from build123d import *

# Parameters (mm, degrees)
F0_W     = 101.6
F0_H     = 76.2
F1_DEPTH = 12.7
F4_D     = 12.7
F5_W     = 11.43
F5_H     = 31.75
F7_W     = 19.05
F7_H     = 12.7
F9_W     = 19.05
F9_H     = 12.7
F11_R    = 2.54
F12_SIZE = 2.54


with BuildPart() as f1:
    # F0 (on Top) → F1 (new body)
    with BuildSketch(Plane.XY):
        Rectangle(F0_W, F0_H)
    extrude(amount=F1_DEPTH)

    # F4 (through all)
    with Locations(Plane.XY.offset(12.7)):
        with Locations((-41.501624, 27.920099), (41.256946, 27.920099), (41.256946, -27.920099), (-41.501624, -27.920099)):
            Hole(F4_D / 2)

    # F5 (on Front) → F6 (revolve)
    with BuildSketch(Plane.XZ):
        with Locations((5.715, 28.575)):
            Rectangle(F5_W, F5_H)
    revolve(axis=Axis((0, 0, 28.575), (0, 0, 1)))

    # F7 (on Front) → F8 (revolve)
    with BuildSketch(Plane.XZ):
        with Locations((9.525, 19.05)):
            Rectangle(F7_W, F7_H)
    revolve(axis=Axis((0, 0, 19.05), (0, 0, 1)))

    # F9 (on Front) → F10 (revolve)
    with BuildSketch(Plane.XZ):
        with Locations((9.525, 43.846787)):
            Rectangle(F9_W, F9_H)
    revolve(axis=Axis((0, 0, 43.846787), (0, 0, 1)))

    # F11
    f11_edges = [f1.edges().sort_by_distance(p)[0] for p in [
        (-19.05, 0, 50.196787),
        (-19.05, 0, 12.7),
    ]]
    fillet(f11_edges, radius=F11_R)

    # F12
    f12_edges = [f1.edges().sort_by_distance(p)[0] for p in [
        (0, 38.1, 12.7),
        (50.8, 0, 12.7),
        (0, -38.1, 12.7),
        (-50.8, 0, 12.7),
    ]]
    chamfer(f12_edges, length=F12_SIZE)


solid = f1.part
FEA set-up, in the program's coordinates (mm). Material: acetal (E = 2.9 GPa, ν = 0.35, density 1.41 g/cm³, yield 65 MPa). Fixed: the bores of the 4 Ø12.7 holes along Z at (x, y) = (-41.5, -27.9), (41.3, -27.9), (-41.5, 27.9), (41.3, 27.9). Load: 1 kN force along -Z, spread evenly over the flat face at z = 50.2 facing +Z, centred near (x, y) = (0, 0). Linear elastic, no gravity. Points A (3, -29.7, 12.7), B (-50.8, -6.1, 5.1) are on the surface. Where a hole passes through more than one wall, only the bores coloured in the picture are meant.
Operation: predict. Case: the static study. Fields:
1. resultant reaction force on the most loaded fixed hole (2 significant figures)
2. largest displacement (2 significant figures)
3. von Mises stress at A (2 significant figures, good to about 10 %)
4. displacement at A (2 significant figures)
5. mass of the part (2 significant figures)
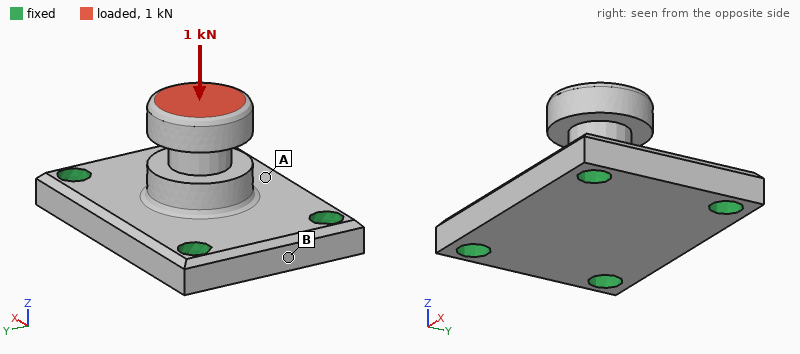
260 N
85 µm
1.8 MPa
49 µm
180 g
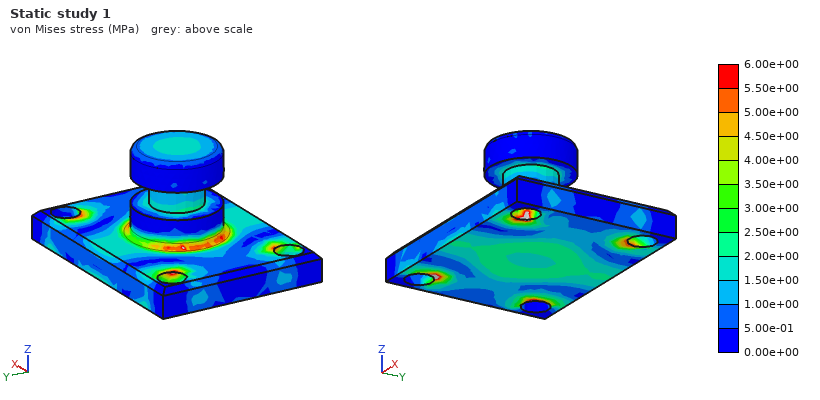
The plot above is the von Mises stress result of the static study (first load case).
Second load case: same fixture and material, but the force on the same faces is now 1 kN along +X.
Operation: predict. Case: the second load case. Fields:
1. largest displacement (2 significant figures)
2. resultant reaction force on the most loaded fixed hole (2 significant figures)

0.49 mm
450 N
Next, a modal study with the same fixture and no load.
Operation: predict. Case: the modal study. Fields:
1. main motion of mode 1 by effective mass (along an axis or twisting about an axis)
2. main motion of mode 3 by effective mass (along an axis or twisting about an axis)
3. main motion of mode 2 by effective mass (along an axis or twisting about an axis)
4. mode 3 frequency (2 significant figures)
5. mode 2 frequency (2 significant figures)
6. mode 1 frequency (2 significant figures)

along Y
along Z
along X
2000 Hz
1900 Hz
1600 Hz
